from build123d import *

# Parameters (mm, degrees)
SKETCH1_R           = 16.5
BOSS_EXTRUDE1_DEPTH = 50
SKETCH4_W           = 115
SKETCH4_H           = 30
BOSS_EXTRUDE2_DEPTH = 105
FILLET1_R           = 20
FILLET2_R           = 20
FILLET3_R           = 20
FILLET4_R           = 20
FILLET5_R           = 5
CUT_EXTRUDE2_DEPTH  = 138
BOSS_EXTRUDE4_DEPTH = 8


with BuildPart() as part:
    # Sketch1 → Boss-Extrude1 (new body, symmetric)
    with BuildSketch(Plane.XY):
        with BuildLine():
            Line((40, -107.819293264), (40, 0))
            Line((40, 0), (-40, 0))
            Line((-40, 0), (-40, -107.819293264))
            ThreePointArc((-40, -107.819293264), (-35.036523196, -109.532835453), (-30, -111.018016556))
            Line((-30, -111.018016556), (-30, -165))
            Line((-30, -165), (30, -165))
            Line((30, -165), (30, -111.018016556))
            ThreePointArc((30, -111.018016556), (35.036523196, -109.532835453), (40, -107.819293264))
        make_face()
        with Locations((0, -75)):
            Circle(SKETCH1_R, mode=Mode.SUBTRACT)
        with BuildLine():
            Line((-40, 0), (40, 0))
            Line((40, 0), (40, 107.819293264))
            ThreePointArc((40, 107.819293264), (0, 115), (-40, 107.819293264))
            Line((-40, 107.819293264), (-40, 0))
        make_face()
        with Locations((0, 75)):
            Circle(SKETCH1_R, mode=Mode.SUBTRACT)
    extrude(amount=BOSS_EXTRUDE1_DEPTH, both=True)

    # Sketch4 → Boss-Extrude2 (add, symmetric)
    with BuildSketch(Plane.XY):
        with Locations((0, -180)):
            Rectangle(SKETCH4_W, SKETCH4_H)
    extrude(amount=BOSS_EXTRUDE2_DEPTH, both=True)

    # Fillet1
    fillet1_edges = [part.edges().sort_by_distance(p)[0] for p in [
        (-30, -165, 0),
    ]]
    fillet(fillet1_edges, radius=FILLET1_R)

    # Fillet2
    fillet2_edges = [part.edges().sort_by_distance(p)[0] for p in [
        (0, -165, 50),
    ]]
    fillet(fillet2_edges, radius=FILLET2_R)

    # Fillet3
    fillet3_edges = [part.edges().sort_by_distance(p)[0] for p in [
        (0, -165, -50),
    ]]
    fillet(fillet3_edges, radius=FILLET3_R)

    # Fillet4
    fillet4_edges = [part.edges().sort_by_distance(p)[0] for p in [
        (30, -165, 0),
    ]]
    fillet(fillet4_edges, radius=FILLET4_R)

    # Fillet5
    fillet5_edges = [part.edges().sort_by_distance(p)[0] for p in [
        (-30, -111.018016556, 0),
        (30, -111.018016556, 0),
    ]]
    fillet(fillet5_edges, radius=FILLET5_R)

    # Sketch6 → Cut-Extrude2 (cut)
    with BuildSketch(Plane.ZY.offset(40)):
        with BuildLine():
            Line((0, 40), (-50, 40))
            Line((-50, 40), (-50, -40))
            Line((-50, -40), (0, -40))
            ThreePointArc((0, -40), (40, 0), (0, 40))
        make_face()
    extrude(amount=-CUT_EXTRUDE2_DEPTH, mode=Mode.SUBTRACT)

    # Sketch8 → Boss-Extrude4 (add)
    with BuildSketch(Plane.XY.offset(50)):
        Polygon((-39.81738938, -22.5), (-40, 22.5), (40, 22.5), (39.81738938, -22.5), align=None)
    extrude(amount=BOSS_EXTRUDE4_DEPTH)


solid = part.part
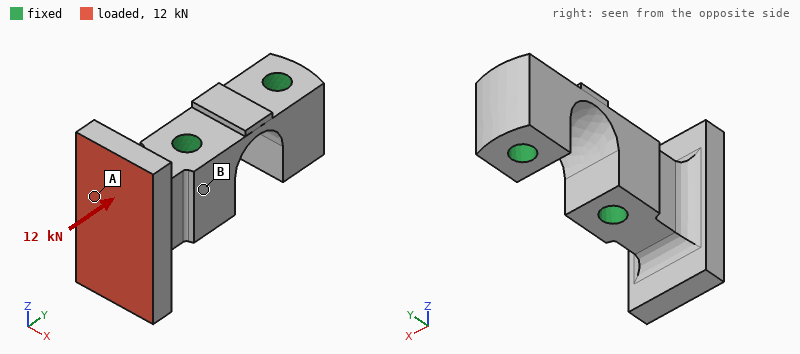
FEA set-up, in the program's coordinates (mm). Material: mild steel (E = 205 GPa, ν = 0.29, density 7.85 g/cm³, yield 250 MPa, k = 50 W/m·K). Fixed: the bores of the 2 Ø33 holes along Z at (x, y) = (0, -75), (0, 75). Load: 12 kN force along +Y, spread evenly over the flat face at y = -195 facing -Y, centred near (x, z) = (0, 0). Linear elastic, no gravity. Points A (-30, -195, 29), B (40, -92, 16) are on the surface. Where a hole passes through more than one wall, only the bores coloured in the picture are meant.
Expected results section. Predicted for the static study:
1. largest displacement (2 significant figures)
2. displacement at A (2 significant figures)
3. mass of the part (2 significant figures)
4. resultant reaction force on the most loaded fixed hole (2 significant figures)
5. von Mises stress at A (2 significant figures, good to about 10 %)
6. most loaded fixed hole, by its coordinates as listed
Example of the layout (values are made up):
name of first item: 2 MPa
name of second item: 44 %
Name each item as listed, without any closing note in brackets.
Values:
largest displacement: 4.1 µm
displacement at A: 0.90 µm
mass of the part: 17 kg
resultant reaction force on the most loaded fixed hole: 12 kN
von Mises stress at A: 3.0 MPa
most loaded fixed hole, by its coordinates as listed: (0, -75)
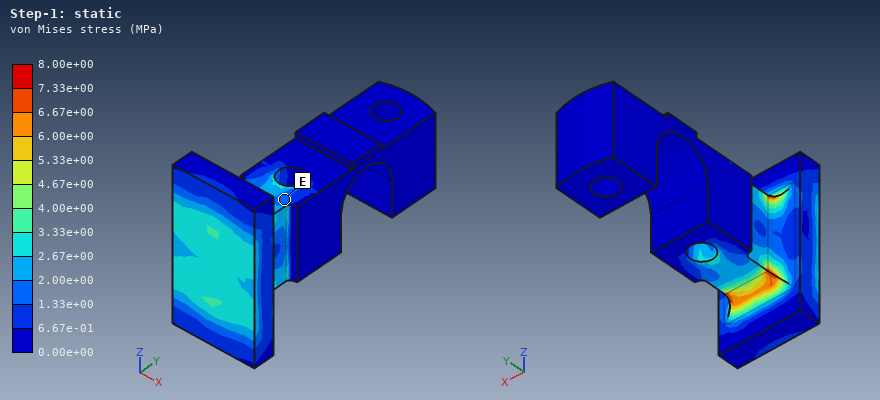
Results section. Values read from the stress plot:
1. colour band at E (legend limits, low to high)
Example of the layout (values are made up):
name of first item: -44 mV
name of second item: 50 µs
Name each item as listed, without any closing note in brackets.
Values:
colour band at E: 1.33e+00 to 2.00e+00 MPa
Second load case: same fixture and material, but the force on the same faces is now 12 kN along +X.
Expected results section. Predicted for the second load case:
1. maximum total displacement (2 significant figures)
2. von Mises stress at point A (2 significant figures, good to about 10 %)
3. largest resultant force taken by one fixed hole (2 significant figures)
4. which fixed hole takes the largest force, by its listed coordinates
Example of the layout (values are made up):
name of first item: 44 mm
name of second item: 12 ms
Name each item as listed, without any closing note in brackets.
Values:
maximum total displacement: 22 µm
von Mises stress at point A: 2.3 MPa
largest resultant force taken by one fixed hole: 13 kN
which fixed hole takes the largest force, by its listed coordinates: (0, -75)
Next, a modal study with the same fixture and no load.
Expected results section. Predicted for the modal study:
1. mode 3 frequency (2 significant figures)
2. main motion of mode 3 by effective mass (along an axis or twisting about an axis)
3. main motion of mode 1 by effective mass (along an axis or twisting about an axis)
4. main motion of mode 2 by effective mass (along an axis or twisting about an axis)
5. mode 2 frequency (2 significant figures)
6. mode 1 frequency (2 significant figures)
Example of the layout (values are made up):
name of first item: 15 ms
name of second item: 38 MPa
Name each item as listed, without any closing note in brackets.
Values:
mode 3 frequency: 2400 Hz
main motion of mode 3 by effective mass: along Z
main motion of mode 1 by effective mass: along X
main motion of mode 2 by effective mass: twisting about Y
mode 2 frequency: 2200 Hz
mode 1 frequency: 1800 Hz
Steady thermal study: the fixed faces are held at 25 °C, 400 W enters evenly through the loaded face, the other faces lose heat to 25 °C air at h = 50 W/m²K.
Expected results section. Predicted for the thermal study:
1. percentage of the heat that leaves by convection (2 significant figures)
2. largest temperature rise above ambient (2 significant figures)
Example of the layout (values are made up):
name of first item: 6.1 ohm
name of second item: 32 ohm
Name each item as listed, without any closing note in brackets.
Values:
percentage of the heat that leaves by convection: 42 %
largest temperature rise above ambient: 82 K
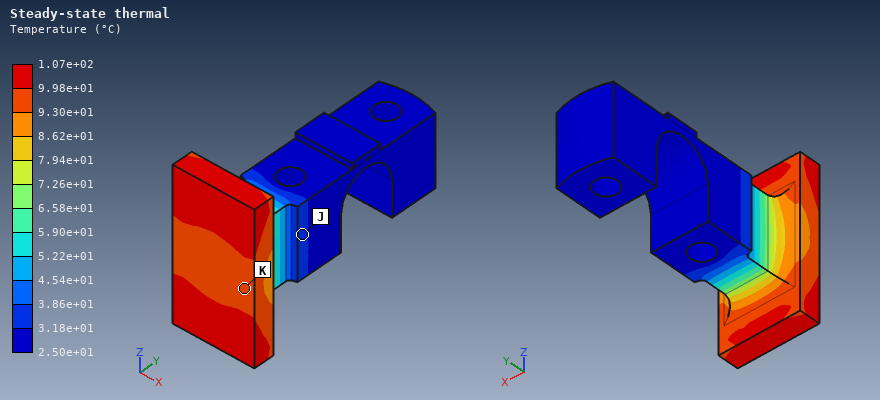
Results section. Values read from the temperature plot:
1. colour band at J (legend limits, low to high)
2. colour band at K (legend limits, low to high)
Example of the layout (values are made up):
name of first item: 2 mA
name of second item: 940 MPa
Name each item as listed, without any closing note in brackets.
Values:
colour band at J: 3.18e+01 to 3.86e+01 °C
colour band at K: 9.30e+01 to 9.98e+01 °C
